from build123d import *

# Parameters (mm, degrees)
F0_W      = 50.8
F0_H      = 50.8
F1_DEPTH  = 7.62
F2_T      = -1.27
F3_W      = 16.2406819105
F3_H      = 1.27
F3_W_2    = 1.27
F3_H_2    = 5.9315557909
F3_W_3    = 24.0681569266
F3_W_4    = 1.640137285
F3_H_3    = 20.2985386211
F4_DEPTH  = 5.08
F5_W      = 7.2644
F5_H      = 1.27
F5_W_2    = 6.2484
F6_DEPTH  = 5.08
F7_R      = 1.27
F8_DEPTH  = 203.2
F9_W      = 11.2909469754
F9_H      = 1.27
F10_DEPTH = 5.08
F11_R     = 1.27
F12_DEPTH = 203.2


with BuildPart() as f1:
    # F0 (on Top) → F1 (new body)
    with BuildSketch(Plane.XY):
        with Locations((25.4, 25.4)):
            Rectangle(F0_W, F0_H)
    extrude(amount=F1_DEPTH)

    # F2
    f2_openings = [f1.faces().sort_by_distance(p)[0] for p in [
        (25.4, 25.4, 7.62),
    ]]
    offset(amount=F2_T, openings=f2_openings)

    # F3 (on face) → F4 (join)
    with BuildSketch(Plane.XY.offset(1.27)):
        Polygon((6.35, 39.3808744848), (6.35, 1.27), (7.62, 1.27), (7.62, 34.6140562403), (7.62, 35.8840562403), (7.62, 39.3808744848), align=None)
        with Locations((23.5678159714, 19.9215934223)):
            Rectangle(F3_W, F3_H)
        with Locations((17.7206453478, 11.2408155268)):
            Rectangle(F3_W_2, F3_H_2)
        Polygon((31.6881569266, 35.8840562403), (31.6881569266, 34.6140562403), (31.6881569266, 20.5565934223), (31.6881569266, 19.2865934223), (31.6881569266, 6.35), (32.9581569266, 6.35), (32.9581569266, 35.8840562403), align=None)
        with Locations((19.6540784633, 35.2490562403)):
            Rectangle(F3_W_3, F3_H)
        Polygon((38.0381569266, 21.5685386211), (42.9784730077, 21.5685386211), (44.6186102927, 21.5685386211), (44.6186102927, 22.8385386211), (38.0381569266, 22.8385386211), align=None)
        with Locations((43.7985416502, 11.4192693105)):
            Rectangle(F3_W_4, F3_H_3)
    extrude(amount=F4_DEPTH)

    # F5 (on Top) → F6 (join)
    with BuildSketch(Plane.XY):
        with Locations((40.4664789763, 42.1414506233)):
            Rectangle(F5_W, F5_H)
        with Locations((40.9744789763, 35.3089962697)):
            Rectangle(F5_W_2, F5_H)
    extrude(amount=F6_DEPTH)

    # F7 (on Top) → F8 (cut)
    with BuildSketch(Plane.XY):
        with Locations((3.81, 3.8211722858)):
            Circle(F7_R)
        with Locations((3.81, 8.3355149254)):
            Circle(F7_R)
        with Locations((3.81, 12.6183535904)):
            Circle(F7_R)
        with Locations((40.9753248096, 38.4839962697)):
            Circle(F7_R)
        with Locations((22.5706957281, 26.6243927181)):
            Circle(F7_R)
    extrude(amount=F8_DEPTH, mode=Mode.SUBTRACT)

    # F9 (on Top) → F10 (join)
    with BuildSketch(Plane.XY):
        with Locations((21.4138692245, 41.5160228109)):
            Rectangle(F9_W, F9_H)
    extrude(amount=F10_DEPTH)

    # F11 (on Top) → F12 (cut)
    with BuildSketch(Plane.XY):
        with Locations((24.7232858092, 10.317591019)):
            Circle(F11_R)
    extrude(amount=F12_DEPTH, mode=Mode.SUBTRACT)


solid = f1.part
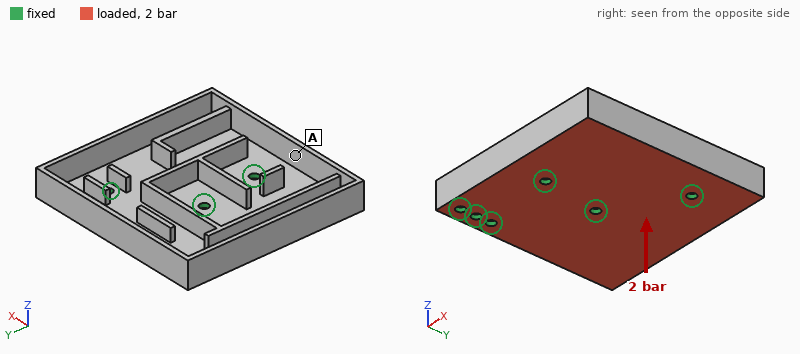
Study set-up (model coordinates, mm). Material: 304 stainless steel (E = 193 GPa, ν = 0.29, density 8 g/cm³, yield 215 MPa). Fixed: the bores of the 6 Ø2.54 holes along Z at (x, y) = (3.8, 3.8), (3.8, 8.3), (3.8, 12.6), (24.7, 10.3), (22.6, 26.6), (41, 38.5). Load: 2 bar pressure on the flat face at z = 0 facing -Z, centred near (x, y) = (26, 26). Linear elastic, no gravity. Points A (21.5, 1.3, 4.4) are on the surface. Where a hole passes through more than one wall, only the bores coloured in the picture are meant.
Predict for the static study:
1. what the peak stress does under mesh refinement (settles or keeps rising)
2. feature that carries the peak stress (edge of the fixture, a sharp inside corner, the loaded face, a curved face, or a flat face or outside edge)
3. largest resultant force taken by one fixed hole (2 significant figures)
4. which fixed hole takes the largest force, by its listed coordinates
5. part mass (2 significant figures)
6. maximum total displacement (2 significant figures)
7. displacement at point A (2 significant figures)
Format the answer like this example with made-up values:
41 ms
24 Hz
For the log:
keeps rising
edge of the fixture
240 N
(3.8, 12.6)
47 g
53 µm
13 µm
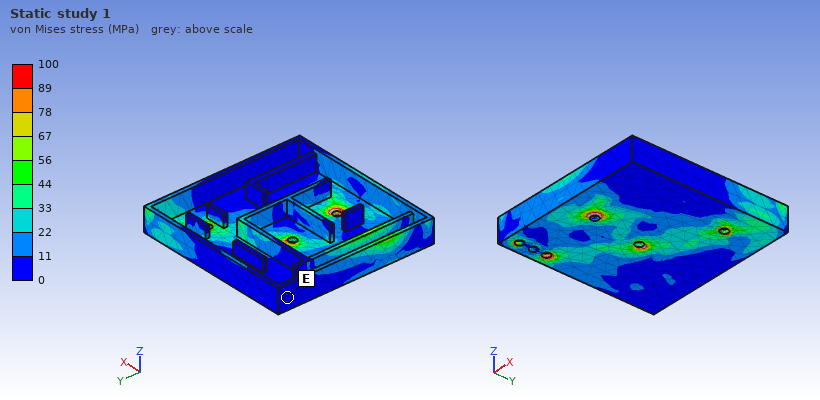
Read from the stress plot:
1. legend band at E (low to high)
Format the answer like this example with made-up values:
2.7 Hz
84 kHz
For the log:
0 to 11 MPa
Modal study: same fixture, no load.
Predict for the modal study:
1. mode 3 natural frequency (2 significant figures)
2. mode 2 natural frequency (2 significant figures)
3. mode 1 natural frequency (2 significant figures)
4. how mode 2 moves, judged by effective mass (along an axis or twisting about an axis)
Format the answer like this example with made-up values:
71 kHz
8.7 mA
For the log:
5200 Hz
2800 Hz
2500 Hz
along Z
